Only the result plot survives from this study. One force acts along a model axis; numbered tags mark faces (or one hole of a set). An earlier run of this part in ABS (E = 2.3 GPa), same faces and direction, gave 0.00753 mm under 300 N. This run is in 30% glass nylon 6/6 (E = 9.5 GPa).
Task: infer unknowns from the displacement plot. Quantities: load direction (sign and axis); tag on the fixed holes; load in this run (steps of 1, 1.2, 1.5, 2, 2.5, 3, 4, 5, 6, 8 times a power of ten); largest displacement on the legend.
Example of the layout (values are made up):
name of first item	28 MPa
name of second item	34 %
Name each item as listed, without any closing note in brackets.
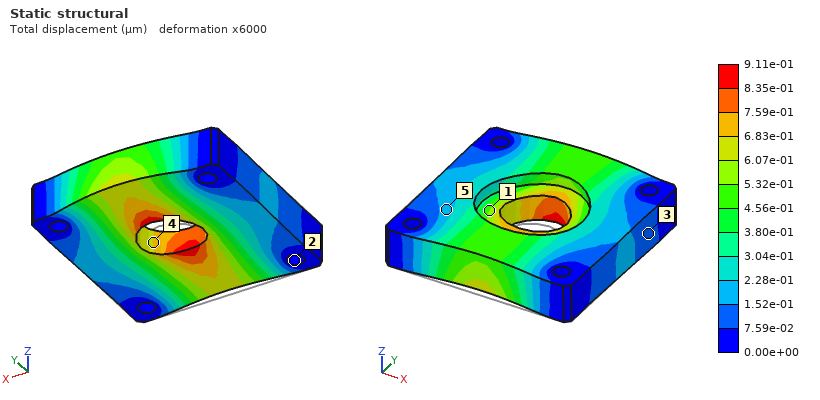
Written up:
load direction	+Y
tag on the fixed holes	2
load in this run	150 N
largest displacement on the legend	9.11e-01 µm
